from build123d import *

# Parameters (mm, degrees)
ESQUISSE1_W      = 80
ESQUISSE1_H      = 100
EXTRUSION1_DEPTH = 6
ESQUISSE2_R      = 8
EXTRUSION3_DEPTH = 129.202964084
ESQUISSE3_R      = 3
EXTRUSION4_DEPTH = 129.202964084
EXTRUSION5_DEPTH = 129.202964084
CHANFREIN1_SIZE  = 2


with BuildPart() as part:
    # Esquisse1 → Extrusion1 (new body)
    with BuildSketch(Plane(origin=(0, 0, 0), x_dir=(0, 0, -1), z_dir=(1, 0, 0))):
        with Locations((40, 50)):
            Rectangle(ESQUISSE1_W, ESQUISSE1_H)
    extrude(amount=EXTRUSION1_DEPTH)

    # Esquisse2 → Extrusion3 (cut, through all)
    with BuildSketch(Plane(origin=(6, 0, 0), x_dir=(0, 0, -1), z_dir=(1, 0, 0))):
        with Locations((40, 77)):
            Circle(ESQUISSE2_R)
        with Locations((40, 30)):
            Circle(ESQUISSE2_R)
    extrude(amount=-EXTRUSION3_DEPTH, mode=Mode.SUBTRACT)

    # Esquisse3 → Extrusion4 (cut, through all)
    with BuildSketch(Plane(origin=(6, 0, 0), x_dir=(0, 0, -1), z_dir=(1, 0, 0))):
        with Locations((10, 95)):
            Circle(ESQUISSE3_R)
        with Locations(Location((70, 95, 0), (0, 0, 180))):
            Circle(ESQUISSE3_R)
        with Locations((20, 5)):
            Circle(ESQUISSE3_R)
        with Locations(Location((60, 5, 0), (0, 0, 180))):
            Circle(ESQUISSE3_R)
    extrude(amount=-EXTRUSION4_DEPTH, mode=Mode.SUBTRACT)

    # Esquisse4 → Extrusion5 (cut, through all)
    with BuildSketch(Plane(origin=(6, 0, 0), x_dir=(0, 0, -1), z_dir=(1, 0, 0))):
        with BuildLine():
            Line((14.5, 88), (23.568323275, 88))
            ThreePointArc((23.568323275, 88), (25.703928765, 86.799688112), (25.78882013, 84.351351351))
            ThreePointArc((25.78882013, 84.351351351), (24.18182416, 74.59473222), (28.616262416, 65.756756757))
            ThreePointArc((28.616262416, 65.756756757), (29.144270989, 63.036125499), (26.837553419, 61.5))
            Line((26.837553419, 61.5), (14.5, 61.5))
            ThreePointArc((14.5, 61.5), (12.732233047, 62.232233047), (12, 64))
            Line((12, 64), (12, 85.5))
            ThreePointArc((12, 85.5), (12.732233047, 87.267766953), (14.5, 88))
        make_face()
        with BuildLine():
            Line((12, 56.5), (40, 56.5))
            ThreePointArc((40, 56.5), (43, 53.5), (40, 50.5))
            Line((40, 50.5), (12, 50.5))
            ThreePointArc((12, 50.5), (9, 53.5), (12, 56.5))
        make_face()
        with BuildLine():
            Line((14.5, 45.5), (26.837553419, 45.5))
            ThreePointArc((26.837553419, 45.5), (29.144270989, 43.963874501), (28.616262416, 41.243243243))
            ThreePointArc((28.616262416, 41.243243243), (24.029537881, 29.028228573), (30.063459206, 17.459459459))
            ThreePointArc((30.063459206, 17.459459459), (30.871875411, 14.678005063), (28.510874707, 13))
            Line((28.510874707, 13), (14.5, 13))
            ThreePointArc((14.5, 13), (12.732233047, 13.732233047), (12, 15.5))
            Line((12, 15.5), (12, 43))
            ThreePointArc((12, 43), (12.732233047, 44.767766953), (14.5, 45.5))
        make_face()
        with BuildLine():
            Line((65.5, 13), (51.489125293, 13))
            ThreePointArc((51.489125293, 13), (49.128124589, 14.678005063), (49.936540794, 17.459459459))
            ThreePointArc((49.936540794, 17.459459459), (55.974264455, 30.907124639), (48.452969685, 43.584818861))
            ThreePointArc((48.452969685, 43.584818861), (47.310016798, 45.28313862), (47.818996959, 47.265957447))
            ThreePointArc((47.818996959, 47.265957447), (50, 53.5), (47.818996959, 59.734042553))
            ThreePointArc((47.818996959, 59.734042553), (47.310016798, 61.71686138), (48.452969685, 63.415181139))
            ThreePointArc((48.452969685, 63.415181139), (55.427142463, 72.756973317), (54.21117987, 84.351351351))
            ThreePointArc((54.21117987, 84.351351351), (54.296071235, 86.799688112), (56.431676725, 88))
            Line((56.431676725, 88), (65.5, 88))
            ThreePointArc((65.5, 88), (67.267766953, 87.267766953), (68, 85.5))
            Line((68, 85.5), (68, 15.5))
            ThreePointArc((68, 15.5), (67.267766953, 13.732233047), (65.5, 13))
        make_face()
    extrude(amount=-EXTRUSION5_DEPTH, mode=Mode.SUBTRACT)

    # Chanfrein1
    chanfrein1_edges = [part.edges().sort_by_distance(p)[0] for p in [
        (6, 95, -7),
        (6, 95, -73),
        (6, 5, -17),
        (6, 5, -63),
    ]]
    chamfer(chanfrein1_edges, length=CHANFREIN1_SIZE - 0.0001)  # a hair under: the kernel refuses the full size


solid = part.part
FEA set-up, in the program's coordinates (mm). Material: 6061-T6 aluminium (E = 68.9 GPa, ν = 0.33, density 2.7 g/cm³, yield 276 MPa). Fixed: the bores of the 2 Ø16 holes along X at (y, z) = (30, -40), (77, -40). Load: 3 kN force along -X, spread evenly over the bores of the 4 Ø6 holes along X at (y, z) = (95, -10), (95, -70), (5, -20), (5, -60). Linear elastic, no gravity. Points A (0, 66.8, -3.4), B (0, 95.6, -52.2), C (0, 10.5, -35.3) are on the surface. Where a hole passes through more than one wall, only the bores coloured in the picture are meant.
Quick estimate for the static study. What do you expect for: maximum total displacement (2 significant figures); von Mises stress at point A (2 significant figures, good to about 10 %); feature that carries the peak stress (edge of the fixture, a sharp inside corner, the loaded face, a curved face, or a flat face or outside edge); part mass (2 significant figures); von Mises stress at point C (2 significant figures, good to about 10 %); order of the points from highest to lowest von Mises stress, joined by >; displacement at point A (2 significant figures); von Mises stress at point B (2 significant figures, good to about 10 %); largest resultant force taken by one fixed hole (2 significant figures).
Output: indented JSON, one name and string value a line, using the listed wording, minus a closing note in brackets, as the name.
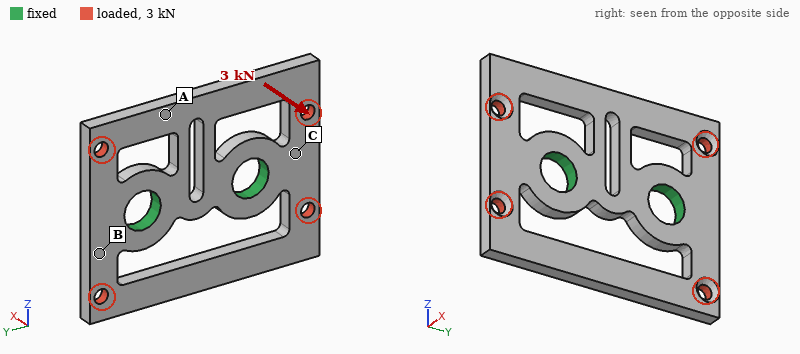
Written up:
{
  "maximum total displacement": "0.41 mm",
  "von Mises stress at point A": "33 MPa",
  "feature that carries the peak stress": "a curved face",
  "part mass": "85 g",
  "von Mises stress at point C": "87 MPa",
  "order of the points from highest to lowest von Mises stress, joined by >": "B > C > A",
  "displacement at point A": "0.16 mm",
  "von Mises stress at point B": "130 MPa",
  "largest resultant force taken by one fixed hole": "1.5 kN"
}
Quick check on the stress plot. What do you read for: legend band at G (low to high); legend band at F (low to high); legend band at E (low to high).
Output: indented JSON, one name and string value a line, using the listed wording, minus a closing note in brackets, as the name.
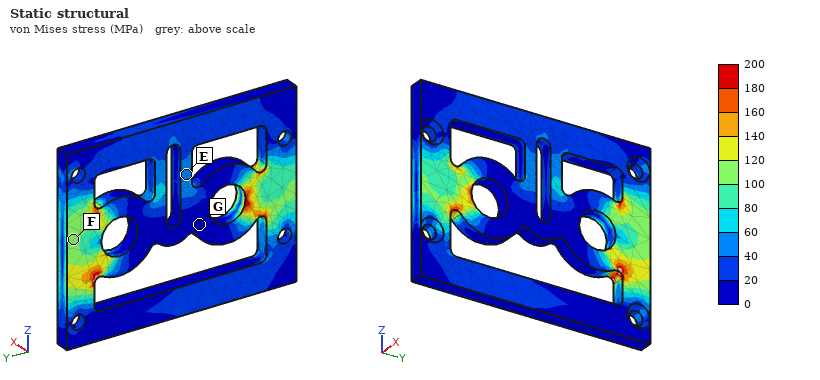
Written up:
{
  "legend band at G": "0 to 20 MPa",
  "legend band at F": "100 to 120 MPa",
  "legend band at E": "40 to 60 MPa"
}
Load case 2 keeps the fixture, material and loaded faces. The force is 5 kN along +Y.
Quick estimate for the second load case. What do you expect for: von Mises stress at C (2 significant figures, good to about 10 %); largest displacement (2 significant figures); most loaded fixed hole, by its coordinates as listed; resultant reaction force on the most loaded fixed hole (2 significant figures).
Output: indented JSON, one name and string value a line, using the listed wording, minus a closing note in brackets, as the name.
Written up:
{
  "von Mises stress at C": "21 MPa",
  "largest displacement": "74 µm",
  "most loaded fixed hole, by its coordinates as listed": "(30, -40)",
  "resultant reaction force on the most loaded fixed hole": "2.7 kN"
}
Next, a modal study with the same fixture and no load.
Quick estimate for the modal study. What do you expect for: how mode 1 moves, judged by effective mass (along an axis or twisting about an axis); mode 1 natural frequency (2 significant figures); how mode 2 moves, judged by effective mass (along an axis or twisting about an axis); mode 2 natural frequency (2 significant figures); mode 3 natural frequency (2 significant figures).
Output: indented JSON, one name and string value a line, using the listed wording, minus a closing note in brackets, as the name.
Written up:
{
  "how mode 1 moves, judged by effective mass": "along X",
  "mode 1 natural frequency": "1500 Hz",
  "how mode 2 moves, judged by effective mass": "along X",
  "mode 2 natural frequency": "2100 Hz",
  "mode 3 natural frequency": "2900 Hz"
}
